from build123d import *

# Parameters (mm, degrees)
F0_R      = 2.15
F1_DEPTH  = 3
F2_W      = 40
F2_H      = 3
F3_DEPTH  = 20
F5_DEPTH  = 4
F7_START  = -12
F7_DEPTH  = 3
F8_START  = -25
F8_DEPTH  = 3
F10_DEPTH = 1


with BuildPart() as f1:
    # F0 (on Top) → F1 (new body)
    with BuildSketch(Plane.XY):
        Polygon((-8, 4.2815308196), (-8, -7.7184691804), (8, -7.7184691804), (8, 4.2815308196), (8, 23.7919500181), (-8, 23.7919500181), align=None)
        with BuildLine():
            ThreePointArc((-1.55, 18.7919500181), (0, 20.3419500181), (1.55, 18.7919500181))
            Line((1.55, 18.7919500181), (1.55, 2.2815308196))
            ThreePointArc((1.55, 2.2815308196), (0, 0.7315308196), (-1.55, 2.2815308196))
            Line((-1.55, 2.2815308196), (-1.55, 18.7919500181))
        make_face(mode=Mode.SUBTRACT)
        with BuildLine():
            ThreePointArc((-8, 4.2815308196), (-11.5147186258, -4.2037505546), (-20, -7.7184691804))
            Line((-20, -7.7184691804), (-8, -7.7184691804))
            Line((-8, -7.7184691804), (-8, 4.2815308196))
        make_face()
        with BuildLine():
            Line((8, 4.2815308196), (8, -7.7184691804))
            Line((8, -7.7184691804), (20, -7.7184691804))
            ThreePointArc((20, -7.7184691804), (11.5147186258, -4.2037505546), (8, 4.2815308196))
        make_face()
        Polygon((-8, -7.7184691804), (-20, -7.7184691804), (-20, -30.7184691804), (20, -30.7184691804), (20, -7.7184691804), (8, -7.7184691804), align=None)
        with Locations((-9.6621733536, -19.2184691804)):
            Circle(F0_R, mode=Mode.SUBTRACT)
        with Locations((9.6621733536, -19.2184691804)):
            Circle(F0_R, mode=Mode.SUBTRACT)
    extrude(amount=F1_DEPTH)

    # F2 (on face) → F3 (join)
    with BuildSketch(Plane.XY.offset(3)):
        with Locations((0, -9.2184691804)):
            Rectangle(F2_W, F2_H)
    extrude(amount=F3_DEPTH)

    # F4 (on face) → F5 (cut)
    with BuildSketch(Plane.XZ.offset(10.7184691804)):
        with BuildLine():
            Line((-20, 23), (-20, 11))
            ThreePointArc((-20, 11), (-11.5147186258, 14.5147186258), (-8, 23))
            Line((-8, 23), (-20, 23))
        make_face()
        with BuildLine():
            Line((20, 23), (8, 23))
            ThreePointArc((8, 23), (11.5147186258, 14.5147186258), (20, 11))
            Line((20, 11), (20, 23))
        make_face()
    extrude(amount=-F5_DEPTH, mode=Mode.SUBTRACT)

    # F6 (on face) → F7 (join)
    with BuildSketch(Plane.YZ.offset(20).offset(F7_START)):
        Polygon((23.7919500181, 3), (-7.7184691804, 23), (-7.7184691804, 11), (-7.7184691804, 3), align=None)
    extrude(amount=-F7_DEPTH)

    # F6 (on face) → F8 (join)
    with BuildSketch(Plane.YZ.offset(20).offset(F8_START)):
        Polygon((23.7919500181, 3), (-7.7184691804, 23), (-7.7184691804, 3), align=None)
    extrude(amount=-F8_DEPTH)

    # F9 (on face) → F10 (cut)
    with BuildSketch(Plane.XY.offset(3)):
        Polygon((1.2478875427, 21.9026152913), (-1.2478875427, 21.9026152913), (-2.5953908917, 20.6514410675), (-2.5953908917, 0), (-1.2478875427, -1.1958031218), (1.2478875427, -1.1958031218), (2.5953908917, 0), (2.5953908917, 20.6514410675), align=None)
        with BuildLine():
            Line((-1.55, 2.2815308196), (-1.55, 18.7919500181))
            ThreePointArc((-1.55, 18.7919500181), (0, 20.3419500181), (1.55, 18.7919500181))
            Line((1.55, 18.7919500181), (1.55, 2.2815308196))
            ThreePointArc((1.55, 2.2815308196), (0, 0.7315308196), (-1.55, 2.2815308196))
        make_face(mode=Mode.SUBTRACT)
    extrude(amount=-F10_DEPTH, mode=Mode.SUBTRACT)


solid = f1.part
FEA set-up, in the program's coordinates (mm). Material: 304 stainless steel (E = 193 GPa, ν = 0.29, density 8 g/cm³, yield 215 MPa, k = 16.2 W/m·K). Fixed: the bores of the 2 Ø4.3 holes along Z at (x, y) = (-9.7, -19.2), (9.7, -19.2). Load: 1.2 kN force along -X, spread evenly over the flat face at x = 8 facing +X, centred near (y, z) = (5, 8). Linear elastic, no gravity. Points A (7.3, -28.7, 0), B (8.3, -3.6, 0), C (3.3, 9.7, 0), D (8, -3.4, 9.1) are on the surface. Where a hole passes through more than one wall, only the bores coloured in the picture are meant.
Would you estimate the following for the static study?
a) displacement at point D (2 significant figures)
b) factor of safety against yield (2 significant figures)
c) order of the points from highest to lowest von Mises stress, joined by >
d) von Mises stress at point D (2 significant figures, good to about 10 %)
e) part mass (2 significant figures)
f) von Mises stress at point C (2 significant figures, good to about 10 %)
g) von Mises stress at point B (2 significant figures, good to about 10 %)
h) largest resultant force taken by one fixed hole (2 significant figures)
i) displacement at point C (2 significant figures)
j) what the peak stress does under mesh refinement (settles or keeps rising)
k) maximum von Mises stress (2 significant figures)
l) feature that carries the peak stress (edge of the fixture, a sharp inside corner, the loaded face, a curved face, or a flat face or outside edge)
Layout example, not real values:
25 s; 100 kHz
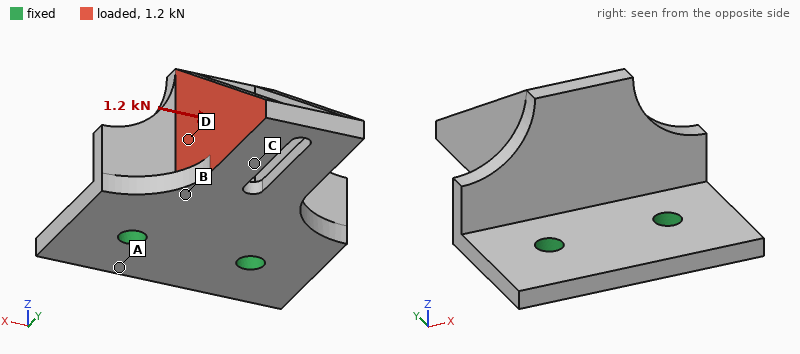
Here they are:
14 µm; 0.79; D > B > C > A; 63 MPa; 62 g; 28 MPa; 49 MPa; 1.5 kN; 14 µm; settles; 270 MPa; a curved face
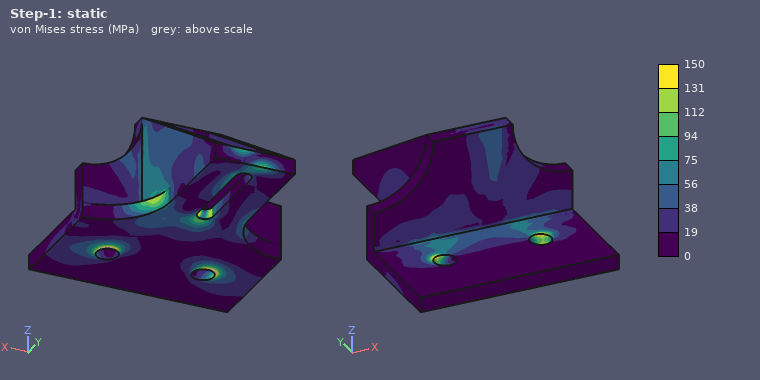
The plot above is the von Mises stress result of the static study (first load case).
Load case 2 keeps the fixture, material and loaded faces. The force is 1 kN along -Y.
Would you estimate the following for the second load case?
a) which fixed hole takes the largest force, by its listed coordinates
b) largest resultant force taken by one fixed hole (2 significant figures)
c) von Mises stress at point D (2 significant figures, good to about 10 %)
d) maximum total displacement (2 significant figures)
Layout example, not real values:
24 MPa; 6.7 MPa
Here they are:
(9.7, -19.2); 890 N; 26 MPa; 0.16 mm
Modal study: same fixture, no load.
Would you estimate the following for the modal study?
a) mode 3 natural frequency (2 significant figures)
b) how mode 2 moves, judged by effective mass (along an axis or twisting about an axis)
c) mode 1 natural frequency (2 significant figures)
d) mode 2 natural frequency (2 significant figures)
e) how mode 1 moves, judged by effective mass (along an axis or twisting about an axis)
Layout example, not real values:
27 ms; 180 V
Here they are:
8000 Hz; along X; 1700 Hz; 6700 Hz; along Z
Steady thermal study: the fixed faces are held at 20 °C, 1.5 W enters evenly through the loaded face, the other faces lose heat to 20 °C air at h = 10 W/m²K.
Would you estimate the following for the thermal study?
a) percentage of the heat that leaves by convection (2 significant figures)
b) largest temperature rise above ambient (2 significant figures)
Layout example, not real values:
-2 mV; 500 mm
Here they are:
27 %; 21 K
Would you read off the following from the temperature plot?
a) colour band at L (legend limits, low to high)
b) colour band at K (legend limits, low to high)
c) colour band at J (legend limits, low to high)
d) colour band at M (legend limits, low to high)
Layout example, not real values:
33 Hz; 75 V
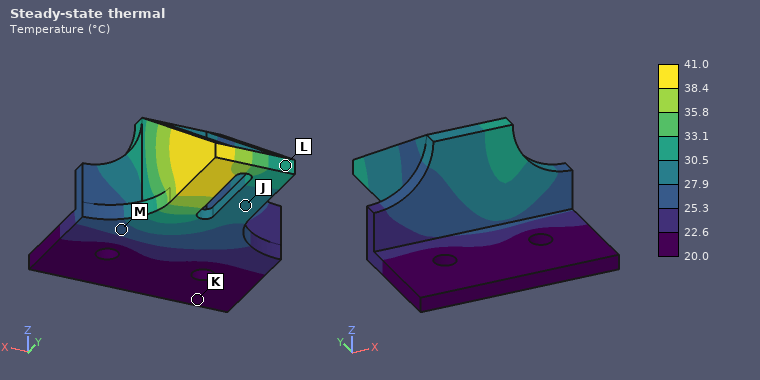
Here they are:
30.5 to 33.1 °C; 20.0 to 22.6 °C; 27.9 to 30.5 °C; 25.3 to 27.9 °C
